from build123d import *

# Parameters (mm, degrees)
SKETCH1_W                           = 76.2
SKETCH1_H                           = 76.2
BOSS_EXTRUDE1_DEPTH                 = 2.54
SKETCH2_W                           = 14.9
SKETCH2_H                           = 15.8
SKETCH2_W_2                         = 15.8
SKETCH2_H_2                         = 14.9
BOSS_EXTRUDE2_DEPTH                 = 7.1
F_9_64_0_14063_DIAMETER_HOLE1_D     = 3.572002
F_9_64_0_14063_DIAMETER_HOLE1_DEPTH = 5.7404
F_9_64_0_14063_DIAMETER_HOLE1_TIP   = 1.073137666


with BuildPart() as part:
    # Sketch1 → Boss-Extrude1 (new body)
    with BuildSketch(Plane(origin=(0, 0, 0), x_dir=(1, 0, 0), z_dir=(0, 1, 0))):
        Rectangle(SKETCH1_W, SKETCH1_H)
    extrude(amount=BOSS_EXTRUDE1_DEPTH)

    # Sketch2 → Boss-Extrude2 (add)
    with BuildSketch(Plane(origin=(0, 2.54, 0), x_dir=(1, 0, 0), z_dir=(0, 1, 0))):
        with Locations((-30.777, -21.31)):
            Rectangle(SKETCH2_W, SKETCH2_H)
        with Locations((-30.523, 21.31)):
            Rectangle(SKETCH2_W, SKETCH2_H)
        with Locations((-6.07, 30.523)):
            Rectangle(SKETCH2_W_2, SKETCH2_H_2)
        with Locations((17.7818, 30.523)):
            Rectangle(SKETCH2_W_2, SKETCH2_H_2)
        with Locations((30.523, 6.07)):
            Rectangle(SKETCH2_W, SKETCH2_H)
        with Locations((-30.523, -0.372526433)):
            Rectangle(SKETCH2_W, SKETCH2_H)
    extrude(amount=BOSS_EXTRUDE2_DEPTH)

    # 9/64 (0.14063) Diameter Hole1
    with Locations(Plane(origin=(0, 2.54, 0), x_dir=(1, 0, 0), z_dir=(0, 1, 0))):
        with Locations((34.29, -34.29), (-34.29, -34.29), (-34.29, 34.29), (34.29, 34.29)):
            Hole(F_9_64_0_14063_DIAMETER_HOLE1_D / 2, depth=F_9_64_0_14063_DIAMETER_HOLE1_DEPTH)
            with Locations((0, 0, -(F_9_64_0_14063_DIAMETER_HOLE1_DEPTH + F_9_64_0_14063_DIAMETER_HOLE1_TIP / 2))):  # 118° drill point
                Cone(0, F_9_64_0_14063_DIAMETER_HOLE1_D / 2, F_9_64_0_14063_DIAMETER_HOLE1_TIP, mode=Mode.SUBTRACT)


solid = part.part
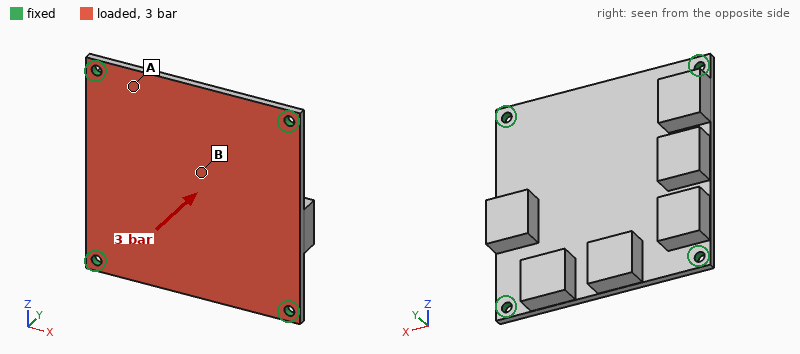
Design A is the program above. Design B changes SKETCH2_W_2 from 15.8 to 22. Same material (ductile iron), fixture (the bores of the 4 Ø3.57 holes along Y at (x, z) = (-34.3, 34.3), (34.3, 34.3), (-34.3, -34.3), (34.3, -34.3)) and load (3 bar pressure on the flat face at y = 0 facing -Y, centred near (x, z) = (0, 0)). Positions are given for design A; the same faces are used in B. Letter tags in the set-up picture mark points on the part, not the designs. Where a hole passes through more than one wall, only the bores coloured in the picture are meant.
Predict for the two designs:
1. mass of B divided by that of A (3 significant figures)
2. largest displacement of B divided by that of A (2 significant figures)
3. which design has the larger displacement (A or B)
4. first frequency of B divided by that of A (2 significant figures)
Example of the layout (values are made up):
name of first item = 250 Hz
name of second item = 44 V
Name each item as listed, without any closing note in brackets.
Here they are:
mass of B divided by that of A = 1.05
largest displacement of B divided by that of A = 0.91
which design has the larger displacement = A
first frequency of B divided by that of A = 1.0
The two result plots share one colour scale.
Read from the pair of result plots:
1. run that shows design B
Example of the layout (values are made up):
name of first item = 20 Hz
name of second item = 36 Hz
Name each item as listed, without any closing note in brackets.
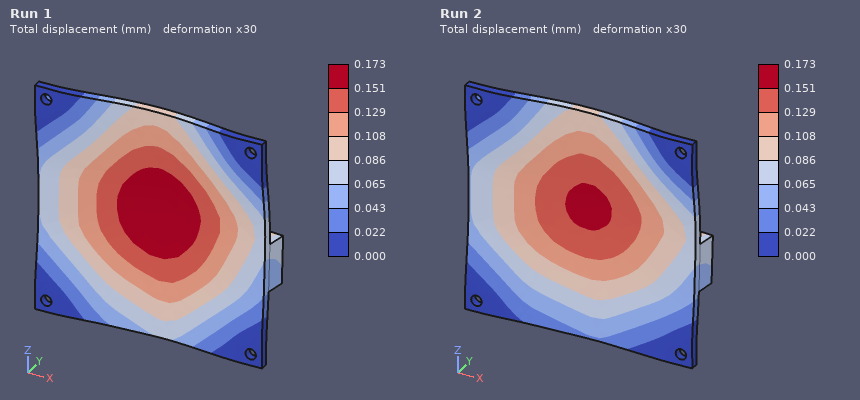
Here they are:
run that shows design B = Run 2
